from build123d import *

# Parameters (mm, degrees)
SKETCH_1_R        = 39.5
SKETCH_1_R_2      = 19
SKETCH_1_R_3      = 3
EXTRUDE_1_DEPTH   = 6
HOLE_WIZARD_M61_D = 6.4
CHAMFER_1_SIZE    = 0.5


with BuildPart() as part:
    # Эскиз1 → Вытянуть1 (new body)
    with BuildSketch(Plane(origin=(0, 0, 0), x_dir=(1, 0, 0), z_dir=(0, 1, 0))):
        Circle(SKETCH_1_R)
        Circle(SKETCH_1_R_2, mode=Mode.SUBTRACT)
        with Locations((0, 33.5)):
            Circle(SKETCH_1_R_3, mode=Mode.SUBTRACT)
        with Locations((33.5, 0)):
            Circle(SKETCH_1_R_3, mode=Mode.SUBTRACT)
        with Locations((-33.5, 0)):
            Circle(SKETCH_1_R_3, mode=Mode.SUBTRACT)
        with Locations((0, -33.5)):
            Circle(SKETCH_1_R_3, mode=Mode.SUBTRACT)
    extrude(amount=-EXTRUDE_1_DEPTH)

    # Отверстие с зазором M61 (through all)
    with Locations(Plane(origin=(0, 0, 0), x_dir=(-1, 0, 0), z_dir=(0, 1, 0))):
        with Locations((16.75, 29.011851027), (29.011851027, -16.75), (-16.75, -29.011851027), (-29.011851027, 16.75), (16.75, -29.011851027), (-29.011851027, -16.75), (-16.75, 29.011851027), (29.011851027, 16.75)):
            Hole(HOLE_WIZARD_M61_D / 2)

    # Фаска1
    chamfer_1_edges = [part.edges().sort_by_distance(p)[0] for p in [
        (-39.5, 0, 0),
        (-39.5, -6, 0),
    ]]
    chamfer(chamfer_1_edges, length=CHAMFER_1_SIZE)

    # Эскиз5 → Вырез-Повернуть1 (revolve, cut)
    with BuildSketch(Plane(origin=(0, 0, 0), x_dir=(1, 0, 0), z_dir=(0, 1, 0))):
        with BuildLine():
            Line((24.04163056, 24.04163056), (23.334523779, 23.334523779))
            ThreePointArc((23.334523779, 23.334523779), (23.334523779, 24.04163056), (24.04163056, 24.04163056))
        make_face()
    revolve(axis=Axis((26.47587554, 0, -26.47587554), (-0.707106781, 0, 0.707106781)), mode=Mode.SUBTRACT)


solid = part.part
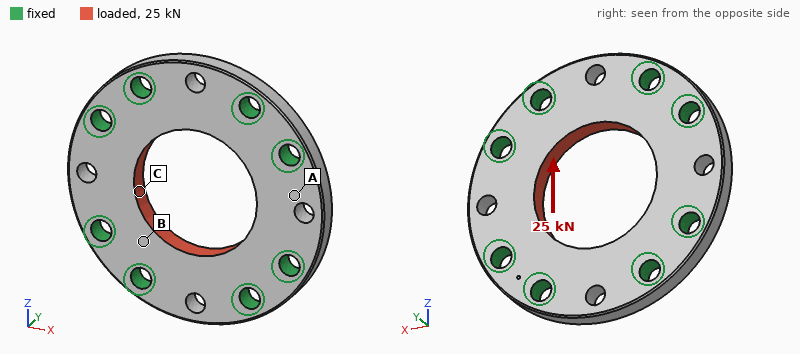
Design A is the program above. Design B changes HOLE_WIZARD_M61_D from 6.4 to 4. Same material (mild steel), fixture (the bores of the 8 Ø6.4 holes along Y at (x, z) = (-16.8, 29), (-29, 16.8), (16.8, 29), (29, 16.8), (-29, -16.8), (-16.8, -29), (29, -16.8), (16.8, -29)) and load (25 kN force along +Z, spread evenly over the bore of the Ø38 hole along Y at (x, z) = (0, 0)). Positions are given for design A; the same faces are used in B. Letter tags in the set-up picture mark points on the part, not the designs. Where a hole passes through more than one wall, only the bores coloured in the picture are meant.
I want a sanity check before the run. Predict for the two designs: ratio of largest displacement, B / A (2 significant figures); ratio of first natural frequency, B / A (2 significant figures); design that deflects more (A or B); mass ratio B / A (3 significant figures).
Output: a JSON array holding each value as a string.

["1.2", "0.82", "B", "1.05"]
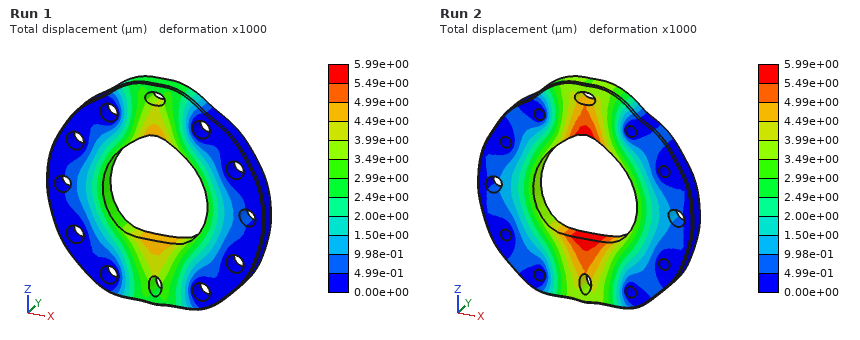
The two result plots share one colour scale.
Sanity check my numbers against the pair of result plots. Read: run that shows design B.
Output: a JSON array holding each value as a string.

["Run 2"]
